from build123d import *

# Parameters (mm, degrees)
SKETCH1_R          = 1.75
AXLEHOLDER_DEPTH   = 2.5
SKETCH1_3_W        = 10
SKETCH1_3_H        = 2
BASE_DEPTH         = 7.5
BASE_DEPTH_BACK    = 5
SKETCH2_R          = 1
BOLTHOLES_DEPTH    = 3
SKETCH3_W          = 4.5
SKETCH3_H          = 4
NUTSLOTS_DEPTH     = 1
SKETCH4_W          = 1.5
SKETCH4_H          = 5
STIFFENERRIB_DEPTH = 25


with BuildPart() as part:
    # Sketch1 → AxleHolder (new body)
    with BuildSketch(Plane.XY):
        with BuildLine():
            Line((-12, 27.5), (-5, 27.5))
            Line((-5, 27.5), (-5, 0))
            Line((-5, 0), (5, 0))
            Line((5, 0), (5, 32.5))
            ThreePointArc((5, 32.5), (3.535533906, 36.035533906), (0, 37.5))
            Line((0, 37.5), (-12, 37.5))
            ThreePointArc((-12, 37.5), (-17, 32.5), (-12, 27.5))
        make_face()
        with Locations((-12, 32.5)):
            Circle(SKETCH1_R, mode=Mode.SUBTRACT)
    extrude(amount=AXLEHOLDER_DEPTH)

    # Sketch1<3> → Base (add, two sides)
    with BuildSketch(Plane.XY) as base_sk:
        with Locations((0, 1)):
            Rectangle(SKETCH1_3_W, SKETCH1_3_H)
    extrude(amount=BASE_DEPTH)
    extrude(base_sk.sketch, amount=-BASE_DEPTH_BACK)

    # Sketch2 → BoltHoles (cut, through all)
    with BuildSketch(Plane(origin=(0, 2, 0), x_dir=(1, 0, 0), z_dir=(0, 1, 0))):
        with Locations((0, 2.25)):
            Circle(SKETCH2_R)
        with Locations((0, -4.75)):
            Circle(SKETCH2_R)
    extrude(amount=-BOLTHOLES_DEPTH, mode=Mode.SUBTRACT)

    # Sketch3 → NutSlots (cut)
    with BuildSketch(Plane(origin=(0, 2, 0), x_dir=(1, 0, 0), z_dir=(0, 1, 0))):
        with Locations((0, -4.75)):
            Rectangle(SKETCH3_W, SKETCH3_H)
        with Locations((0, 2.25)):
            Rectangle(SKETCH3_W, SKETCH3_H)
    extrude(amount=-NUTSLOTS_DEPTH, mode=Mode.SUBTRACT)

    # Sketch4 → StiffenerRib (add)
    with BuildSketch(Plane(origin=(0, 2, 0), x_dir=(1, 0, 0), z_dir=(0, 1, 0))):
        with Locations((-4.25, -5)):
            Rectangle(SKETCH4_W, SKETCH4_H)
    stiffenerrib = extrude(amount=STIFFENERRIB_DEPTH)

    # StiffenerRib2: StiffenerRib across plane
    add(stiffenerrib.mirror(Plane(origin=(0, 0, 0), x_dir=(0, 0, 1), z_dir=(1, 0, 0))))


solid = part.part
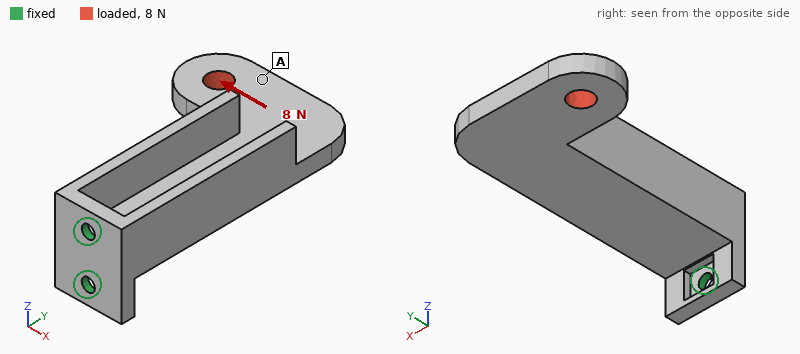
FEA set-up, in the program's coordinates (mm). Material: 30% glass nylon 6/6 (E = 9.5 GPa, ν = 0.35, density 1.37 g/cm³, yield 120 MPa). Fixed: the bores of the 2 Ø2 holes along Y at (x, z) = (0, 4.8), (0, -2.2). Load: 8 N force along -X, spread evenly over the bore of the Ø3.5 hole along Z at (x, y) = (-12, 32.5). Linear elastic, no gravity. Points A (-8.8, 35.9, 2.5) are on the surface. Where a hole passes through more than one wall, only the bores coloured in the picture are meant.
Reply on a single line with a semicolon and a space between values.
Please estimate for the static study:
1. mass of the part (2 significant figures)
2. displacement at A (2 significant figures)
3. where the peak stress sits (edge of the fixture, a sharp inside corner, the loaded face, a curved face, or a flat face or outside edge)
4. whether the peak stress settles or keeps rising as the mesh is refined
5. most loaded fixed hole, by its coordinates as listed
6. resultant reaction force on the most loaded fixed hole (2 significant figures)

2.3 g; 0.34 mm; edge of the fixture; keeps rising; (0, -2.2); 5.0 N
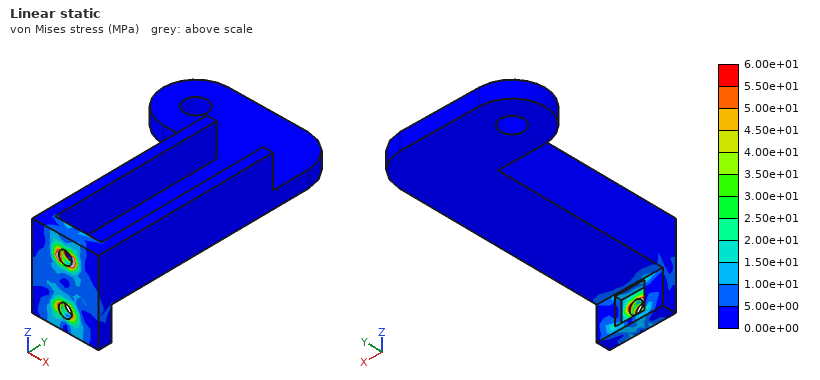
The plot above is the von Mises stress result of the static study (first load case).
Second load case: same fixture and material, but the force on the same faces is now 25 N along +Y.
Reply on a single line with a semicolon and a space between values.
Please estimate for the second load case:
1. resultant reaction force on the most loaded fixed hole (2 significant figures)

14 N
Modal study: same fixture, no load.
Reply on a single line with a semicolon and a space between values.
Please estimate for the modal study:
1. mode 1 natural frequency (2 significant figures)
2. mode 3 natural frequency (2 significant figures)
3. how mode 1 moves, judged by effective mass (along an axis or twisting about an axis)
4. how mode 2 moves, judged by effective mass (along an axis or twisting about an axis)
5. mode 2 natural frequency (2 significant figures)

800 Hz; 2400 Hz; along X; along Z; 1100 Hz
